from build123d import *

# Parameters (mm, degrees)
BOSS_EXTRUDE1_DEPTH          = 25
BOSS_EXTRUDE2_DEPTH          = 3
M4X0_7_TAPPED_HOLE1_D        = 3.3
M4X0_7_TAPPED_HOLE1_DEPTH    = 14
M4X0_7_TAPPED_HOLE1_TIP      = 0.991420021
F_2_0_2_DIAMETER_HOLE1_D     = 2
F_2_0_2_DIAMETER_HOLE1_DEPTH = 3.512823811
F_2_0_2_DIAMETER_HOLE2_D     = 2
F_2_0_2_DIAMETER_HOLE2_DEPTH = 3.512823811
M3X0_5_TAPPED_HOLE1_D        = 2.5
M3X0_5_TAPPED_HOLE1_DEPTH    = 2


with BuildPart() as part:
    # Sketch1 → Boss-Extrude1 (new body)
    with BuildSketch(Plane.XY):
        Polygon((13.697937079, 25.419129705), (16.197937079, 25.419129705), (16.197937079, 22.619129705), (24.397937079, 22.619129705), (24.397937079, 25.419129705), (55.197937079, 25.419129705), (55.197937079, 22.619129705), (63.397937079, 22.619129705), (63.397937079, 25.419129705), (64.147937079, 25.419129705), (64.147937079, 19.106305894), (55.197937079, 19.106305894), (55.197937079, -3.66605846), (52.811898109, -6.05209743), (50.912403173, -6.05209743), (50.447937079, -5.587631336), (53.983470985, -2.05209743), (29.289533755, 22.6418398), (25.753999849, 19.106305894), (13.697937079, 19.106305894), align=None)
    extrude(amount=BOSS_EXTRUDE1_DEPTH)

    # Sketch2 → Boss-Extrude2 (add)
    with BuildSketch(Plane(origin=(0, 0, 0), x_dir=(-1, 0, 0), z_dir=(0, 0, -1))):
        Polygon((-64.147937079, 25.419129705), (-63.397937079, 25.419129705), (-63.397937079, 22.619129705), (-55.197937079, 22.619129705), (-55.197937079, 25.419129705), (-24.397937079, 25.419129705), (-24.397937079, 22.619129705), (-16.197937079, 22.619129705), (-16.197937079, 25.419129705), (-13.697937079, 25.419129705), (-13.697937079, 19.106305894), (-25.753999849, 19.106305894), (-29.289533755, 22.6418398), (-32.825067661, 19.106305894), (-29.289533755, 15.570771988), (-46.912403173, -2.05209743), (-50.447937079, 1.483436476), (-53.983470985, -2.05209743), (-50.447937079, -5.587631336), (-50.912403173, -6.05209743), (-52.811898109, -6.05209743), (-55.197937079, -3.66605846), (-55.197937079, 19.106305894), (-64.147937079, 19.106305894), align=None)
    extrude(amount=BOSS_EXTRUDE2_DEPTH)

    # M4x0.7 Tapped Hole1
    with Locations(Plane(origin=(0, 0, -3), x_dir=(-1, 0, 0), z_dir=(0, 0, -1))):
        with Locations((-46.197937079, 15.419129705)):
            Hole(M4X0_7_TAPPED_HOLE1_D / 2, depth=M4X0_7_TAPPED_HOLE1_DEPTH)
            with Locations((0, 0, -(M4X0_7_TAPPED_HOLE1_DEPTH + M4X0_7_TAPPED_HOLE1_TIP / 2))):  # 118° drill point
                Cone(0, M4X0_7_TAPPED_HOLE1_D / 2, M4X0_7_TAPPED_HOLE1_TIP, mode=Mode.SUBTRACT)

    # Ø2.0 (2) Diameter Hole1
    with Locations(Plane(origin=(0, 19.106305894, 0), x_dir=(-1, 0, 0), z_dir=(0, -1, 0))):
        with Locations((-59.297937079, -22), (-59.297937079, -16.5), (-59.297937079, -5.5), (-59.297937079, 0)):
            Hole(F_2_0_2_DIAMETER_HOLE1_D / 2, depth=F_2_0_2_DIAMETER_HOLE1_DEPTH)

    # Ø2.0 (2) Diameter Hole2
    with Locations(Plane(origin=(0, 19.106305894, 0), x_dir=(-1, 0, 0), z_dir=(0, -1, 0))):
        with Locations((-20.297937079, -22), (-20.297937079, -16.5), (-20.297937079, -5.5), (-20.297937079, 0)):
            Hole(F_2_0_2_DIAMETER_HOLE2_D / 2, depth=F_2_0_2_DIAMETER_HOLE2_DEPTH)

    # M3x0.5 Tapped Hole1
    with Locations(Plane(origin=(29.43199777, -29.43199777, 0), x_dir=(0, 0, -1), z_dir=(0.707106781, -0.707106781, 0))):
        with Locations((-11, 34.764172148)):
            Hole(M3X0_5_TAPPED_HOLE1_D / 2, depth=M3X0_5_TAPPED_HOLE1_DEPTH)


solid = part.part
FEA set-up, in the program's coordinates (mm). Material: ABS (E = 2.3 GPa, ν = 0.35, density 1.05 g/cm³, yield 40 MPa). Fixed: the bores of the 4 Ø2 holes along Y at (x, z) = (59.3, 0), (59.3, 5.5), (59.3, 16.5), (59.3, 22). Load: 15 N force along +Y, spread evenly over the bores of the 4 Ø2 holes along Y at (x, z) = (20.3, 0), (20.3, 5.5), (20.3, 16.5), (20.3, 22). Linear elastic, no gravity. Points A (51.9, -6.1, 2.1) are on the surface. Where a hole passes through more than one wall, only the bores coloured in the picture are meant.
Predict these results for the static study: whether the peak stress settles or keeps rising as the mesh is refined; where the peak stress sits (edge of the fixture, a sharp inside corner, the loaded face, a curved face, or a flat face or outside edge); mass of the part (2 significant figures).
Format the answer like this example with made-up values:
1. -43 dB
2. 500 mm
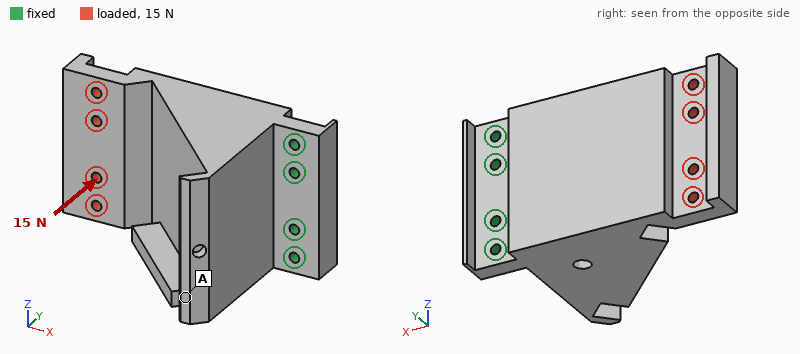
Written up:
1. keeps rising
2. edge of the fixture
3. 15 g
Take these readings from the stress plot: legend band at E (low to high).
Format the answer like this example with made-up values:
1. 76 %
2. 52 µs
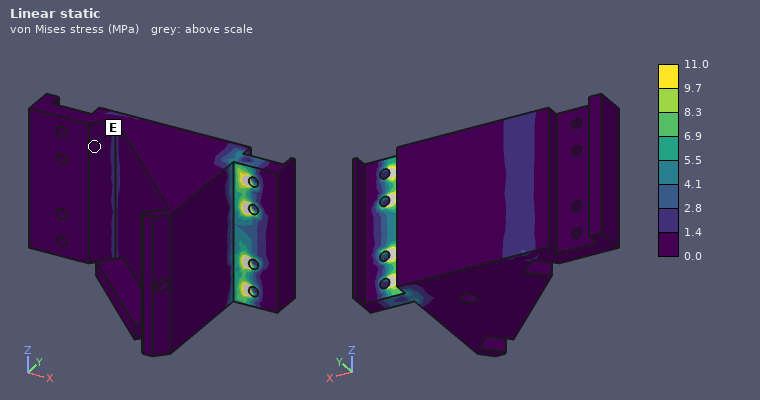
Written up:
1. 0.0 to 1.4 MPa
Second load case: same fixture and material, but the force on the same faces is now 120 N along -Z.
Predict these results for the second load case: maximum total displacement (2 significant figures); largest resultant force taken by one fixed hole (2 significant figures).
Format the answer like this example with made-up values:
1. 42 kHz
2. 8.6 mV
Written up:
1. 0.20 mm
2. 170 N
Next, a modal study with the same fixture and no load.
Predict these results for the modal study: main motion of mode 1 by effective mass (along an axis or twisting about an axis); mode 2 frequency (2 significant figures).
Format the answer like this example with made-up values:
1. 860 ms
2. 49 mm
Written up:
1. along Y
2. 2300 Hz
